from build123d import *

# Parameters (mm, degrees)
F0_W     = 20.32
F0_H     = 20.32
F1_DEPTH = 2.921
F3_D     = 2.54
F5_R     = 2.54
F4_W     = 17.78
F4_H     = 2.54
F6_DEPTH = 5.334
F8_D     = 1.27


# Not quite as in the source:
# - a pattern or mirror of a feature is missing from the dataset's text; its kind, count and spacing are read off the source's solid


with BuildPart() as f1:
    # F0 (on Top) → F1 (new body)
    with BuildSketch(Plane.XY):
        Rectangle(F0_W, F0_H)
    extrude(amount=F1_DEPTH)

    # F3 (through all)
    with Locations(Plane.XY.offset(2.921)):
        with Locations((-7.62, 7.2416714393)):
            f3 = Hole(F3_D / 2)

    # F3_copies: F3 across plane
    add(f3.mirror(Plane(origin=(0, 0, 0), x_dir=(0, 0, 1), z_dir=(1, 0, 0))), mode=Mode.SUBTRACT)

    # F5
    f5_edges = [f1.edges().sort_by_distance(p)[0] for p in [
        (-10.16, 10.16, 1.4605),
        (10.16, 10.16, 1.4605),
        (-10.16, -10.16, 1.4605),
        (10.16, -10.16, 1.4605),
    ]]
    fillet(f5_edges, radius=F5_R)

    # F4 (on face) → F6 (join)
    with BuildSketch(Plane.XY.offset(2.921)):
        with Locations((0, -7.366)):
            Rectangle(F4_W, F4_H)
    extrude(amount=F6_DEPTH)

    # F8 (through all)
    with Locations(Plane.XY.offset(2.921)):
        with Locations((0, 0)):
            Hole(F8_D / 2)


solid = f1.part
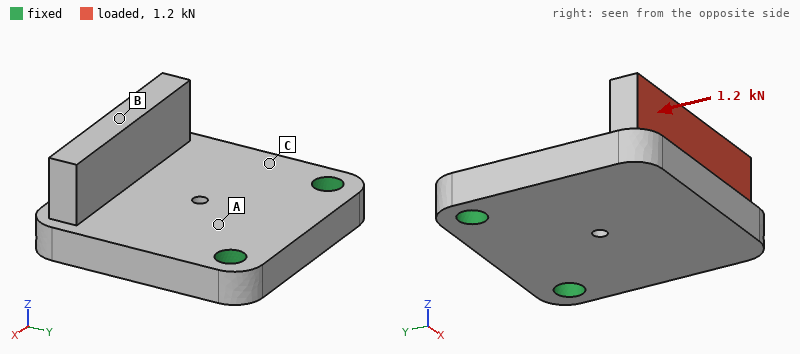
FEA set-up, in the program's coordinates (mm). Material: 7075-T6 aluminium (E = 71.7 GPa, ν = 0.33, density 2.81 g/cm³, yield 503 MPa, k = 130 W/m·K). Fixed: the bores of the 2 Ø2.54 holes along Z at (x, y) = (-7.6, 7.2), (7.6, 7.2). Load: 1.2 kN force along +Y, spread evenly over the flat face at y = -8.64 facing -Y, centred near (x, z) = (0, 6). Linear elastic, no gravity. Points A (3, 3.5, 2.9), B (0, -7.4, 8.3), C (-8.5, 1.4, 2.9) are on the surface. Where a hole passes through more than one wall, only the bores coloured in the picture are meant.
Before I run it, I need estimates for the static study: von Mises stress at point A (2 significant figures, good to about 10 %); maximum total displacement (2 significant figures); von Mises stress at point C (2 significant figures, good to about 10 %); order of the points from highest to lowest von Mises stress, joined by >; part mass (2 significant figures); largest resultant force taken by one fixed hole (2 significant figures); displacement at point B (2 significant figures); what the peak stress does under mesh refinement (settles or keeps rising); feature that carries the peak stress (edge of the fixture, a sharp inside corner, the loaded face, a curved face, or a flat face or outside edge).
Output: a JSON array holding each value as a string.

["150 MPa", "0.28 mm", "210 MPa", "C > A > B", "3.9 g", "620 N", "0.26 mm", "keeps rising", "edge of the fixture"]
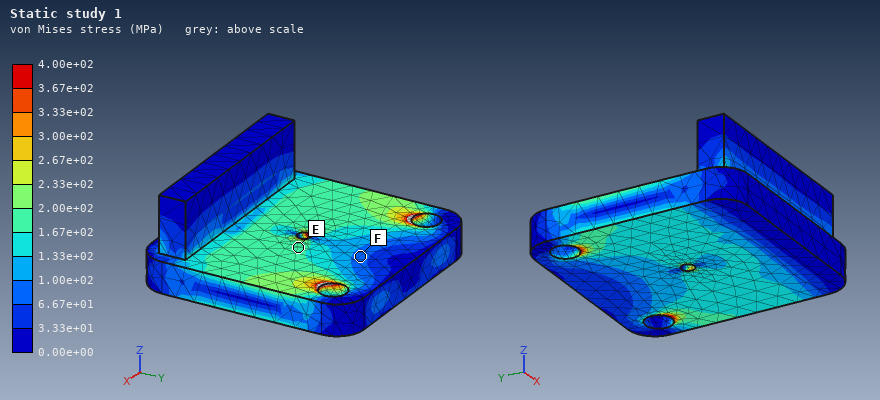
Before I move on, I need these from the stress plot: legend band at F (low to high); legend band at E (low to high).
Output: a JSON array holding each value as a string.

["6.67e+01 to 1.00e+02 MPa", "1.67e+02 to 2.00e+02 MPa"]
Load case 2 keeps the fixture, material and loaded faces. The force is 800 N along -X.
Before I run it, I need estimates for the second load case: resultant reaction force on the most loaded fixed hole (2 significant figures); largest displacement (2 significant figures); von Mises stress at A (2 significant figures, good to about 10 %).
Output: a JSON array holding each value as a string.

["900 N", "75 µm", "73 MPa"]
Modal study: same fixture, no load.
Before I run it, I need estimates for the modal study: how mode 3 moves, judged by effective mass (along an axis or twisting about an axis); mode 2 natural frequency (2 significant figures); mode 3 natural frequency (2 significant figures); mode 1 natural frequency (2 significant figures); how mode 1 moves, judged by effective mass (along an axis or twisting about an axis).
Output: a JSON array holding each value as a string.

["along X", "14 kHz", "27 kHz", "5800 Hz", "along Z"]
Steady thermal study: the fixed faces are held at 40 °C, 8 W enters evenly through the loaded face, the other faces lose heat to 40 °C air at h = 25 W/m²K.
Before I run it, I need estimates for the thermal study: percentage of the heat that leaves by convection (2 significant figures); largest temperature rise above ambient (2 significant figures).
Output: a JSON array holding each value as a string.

["3.4 %", "20 K"]
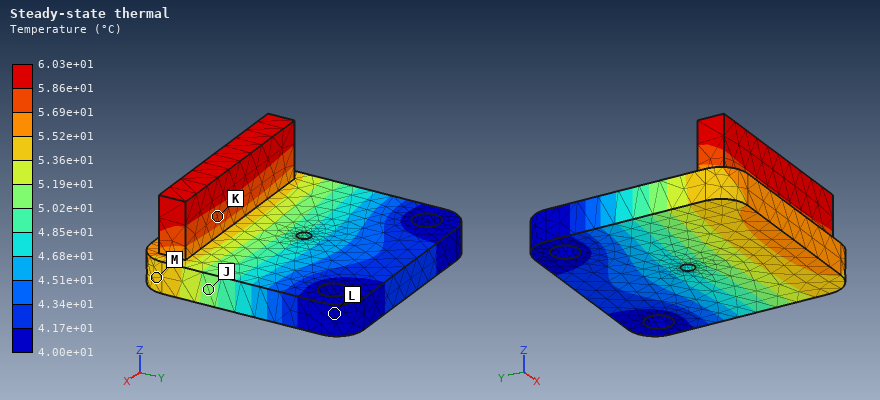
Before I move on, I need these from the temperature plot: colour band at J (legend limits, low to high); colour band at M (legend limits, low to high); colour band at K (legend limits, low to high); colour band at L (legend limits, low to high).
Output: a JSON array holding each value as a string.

["5.02e+01 to 5.19e+01 °C", "5.36e+01 to 5.52e+01 °C", "5.69e+01 to 5.86e+01 °C", "4.00e+01 to 4.17e+01 °C"]
